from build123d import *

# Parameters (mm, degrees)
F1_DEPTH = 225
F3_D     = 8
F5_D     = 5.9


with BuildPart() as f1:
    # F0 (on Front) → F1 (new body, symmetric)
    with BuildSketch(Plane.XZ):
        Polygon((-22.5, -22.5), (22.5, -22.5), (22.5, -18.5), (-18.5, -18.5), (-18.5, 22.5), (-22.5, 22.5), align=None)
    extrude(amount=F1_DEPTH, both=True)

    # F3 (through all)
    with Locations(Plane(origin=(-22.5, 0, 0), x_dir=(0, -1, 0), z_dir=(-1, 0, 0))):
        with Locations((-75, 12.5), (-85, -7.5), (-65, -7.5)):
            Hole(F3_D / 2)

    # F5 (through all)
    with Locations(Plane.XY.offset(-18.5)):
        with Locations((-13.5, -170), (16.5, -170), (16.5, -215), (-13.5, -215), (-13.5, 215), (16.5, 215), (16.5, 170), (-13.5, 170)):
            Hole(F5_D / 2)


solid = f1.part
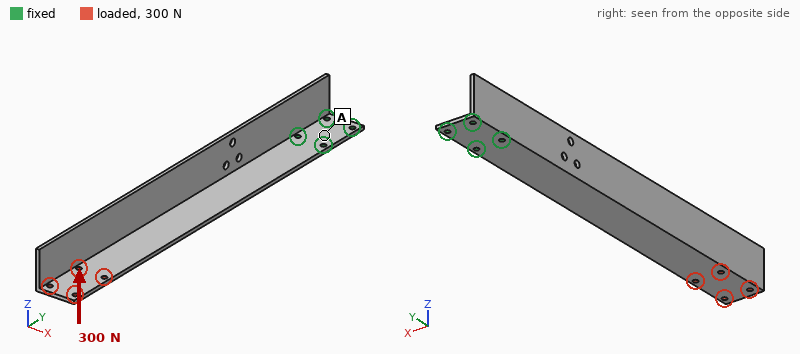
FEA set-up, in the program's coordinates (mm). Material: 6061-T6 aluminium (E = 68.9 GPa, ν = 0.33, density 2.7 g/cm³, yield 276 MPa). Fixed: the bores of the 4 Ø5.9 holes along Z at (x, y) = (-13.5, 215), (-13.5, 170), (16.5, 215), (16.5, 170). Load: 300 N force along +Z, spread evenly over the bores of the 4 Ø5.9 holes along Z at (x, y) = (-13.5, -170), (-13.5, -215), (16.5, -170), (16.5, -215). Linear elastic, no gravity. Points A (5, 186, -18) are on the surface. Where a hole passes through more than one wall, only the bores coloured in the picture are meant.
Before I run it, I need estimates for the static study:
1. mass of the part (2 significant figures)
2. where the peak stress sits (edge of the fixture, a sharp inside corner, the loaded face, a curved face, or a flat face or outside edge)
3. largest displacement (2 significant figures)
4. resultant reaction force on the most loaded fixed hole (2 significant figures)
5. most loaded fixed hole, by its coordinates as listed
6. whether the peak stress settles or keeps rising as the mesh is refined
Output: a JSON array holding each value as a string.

["410 g", "edge of the fixture", "4.8 mm", "3.0 kN", "(-13.5, 170)", "keeps rising"]
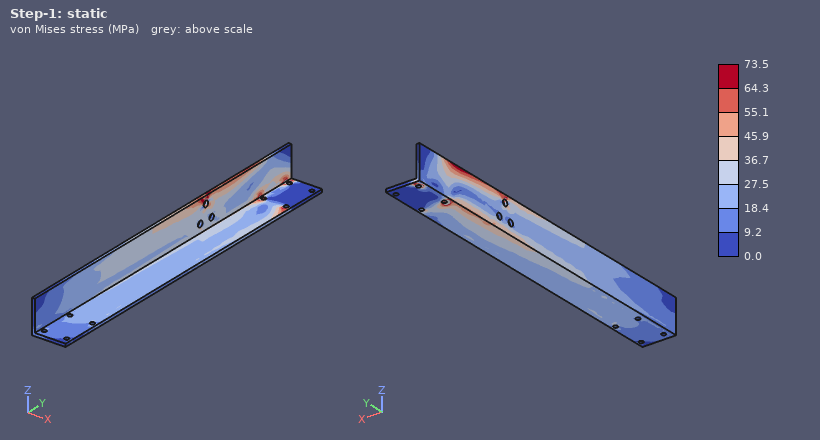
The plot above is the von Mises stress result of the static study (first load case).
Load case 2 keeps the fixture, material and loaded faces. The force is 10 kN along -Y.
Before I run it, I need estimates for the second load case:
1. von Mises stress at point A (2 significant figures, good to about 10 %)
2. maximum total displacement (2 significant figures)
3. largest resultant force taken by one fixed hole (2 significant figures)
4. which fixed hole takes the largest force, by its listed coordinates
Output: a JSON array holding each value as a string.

["11 MPa", "1.7 mm", "4.9 kN", "(16.5, 170)"]
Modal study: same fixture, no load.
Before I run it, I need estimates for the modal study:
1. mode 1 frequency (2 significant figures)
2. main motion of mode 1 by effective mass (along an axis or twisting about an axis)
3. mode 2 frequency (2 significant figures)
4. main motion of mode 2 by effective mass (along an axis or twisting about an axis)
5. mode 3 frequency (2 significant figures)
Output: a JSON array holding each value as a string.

["140 Hz", "along Z", "170 Hz", "along X", "340 Hz"]
